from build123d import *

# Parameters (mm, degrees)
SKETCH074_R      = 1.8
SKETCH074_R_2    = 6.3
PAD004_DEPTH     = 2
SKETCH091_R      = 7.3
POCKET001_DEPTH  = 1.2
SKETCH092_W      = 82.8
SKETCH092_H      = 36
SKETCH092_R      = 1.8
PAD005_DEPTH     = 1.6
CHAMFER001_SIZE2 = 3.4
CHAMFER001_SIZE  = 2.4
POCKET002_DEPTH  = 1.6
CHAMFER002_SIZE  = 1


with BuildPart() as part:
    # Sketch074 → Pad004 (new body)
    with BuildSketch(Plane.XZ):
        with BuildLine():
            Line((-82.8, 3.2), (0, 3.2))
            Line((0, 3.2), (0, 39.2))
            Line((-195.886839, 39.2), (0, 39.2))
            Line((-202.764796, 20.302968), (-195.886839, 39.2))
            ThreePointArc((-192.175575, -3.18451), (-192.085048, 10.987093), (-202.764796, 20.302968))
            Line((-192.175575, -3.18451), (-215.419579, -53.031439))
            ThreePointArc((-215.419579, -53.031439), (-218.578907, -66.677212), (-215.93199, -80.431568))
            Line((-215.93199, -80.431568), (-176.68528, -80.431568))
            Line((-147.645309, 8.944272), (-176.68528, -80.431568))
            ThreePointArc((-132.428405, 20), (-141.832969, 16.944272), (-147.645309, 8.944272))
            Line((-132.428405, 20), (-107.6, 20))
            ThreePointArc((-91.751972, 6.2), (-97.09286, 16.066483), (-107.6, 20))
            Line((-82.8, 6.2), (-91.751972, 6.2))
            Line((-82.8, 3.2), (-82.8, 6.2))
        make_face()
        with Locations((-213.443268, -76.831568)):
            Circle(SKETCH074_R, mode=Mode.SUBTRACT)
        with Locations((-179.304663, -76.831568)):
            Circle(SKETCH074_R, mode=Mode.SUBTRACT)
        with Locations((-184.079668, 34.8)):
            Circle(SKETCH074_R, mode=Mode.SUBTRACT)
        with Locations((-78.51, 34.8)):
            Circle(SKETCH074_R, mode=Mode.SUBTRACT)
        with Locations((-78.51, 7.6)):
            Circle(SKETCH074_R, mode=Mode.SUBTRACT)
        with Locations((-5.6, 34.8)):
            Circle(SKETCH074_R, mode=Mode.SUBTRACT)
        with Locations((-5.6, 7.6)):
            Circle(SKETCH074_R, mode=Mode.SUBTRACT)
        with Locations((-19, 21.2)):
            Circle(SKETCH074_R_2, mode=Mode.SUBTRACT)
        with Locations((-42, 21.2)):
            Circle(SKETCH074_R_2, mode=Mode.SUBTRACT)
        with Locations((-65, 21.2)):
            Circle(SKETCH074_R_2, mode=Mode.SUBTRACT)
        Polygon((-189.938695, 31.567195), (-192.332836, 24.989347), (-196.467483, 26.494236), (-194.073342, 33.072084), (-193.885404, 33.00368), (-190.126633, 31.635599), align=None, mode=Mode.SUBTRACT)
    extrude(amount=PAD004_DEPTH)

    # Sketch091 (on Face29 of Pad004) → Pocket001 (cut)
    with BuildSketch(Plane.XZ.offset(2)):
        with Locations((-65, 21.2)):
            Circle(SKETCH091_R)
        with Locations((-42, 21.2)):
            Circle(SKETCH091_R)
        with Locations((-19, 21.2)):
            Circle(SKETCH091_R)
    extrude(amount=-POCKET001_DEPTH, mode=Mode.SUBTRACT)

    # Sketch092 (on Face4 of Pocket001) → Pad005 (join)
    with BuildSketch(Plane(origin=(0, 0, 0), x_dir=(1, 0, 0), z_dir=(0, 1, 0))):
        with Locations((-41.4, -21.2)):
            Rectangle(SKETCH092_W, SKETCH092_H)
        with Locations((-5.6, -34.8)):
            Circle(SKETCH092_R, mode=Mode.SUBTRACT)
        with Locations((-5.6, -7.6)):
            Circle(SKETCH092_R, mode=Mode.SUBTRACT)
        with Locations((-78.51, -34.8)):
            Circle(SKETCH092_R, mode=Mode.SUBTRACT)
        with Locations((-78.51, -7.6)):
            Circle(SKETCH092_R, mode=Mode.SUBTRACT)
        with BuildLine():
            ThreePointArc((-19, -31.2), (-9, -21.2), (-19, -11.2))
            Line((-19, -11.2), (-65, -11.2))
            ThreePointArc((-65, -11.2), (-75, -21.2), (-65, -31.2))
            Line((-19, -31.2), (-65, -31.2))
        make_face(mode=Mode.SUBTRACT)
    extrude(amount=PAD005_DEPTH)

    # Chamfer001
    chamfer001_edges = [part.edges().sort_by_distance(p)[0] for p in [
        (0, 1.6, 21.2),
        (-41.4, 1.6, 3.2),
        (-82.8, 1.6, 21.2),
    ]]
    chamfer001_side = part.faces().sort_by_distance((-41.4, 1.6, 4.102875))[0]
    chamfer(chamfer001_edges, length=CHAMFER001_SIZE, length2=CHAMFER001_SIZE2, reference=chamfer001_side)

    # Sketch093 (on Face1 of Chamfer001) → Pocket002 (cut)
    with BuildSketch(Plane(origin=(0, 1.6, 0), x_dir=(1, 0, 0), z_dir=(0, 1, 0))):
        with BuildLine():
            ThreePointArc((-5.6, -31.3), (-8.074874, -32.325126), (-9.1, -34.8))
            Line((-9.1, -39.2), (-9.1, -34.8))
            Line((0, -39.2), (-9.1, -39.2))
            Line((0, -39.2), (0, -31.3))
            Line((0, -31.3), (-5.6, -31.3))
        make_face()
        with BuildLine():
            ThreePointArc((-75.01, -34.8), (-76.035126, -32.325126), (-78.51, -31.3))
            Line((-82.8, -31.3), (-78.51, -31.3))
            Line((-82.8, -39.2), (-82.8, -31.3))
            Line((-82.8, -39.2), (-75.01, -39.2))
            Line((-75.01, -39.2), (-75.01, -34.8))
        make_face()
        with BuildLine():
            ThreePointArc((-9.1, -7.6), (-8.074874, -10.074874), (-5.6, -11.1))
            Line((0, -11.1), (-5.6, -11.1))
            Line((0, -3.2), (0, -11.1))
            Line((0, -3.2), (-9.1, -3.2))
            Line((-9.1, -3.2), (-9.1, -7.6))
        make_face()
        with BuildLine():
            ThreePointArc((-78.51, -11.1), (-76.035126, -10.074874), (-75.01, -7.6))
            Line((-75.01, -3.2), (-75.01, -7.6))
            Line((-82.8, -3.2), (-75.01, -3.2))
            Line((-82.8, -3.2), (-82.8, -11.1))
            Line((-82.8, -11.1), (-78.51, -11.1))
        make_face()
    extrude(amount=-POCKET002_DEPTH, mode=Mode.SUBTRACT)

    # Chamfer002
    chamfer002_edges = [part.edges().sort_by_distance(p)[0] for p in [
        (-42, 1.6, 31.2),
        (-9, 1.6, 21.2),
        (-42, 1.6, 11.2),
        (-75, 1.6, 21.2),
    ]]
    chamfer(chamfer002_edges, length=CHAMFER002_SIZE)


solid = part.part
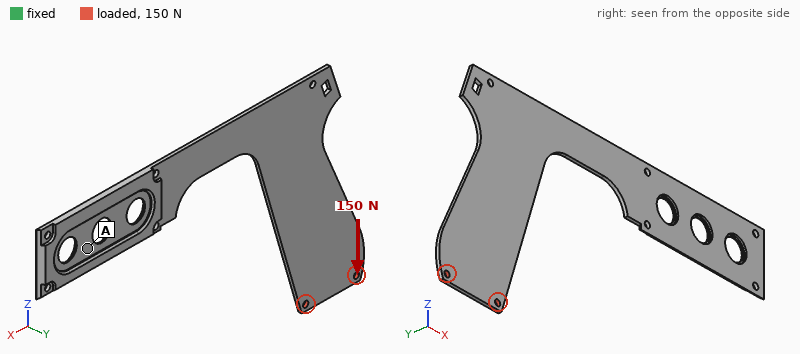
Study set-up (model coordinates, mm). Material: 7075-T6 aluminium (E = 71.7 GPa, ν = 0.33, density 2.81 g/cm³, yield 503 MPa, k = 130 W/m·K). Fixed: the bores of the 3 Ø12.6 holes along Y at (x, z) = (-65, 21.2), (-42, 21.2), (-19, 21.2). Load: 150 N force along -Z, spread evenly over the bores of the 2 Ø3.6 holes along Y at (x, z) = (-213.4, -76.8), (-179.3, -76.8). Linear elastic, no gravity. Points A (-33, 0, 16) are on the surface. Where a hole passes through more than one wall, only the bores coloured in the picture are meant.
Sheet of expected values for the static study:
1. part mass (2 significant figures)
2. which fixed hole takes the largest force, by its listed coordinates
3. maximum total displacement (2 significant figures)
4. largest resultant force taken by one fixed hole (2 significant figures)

58 g
(-65, 21.2)
1.4 mm
490 N
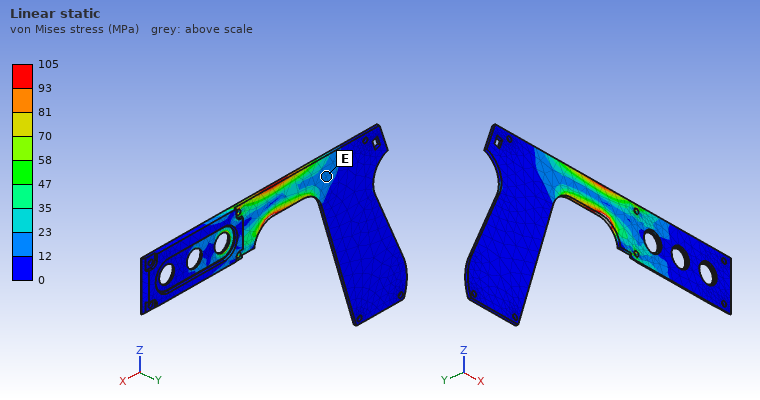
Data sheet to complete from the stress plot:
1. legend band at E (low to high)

12 to 23 MPa
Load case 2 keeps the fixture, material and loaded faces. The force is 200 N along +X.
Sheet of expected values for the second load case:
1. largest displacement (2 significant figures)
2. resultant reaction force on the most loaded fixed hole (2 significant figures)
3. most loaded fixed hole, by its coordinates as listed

2.4 mm
410 N
(-65, 21.2)
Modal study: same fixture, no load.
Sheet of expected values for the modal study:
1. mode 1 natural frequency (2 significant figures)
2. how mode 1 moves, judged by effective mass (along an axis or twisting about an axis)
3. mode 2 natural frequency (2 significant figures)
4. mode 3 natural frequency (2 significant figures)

39 Hz
along Y
130 Hz
370 Hz
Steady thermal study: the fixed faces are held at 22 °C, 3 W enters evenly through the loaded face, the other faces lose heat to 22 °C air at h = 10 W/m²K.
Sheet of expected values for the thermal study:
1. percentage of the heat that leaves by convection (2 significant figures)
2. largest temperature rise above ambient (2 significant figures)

77 %
32 K
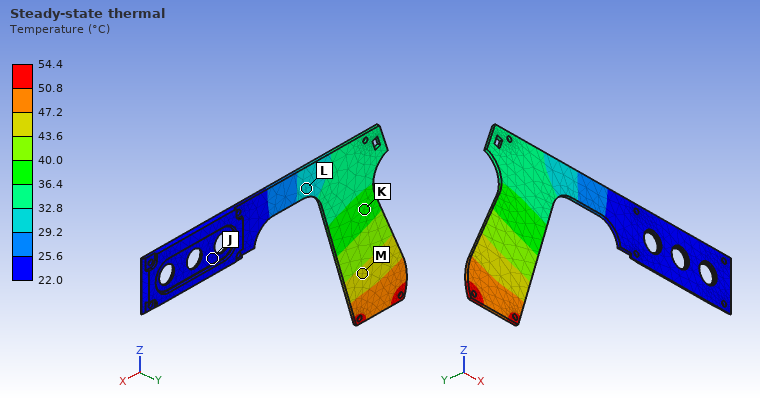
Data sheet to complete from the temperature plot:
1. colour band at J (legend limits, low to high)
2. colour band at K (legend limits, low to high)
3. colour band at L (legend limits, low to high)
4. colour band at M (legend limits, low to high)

22.0 to 25.6 °C
36.4 to 40.0 °C
29.2 to 32.8 °C
43.6 to 47.2 °C
